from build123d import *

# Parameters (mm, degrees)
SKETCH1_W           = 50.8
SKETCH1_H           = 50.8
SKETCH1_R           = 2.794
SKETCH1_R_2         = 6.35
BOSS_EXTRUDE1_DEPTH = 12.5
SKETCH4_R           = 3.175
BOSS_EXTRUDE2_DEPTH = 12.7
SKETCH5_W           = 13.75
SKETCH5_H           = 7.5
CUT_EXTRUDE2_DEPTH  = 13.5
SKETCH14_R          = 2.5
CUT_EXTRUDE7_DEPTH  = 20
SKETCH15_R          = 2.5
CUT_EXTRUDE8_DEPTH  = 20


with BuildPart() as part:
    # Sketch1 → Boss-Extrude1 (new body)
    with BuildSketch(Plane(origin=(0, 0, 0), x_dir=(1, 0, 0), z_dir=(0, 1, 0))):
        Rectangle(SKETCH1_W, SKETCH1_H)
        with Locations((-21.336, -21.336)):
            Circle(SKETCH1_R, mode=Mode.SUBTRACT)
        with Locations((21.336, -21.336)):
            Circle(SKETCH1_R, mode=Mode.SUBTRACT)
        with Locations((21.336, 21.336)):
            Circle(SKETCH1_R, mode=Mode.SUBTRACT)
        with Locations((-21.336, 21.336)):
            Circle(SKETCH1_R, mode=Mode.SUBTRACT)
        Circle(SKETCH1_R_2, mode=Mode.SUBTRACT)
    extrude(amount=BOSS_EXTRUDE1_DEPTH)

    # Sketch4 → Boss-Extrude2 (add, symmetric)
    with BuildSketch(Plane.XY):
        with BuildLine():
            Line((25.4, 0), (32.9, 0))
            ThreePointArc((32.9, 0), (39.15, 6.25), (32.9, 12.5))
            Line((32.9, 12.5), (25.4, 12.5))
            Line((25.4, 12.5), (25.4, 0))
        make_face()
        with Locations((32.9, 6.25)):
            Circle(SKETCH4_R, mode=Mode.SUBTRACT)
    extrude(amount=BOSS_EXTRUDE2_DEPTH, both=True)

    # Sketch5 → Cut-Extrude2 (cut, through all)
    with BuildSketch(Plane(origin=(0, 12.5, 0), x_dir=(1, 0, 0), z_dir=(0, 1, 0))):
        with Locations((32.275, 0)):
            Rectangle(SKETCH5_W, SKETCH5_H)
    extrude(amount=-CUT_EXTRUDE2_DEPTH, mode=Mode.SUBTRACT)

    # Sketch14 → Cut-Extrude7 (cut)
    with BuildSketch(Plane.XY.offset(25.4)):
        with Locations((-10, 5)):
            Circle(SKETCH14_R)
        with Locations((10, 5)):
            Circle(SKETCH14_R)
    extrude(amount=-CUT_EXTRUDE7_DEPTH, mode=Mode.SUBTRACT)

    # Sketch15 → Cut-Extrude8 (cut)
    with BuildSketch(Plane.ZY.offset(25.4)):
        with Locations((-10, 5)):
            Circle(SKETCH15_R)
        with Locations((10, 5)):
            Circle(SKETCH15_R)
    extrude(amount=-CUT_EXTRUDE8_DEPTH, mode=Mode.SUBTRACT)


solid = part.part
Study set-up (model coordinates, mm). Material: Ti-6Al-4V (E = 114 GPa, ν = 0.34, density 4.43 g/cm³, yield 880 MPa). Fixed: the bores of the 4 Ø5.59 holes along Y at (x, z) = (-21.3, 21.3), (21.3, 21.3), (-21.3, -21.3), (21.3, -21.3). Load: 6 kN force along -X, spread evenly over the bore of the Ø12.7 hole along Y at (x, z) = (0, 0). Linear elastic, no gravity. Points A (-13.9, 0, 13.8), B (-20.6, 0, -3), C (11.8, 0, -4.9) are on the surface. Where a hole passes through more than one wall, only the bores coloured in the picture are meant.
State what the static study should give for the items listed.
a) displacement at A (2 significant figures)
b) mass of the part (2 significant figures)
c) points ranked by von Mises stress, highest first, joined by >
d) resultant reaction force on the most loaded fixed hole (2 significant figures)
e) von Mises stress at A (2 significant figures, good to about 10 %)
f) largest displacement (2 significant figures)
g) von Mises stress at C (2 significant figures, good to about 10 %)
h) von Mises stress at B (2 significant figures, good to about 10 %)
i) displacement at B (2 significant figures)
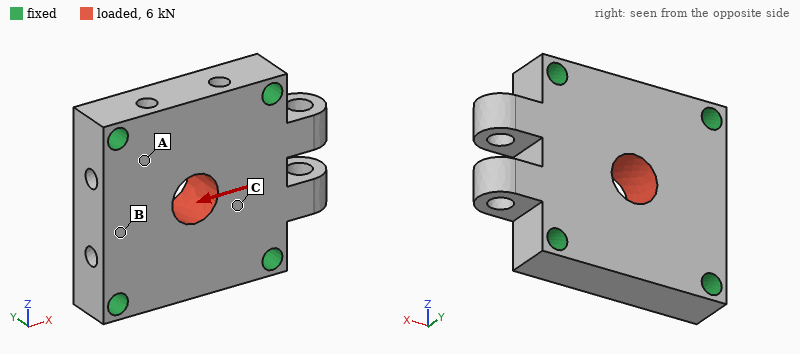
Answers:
1.3 µm
130 g
A > C > B
1.8 kN
13 MPa
3.4 µm
8.9 MPa
3.3 MPa
2.5 µm
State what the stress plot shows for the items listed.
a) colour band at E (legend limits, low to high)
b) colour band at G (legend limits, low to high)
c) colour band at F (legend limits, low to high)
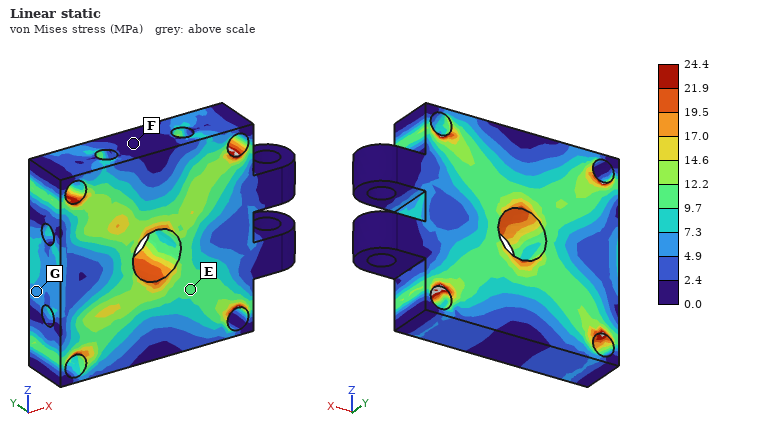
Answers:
9.7 to 12.2 MPa
4.9 to 7.3 MPa
0.0 to 2.4 MPa
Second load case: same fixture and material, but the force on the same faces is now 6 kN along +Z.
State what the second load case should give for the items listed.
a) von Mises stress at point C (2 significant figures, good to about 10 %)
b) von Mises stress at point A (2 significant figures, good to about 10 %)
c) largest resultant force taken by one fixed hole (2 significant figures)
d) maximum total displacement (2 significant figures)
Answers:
10 MPa
13 MPa
1.8 kN
3.4 µm
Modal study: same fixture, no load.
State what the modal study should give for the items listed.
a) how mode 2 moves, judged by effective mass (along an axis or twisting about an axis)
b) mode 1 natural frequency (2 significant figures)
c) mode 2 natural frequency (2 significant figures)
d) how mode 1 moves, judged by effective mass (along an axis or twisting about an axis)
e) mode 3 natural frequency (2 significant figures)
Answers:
along Y
17 kHz
18 kHz
along Y
22 kHz
